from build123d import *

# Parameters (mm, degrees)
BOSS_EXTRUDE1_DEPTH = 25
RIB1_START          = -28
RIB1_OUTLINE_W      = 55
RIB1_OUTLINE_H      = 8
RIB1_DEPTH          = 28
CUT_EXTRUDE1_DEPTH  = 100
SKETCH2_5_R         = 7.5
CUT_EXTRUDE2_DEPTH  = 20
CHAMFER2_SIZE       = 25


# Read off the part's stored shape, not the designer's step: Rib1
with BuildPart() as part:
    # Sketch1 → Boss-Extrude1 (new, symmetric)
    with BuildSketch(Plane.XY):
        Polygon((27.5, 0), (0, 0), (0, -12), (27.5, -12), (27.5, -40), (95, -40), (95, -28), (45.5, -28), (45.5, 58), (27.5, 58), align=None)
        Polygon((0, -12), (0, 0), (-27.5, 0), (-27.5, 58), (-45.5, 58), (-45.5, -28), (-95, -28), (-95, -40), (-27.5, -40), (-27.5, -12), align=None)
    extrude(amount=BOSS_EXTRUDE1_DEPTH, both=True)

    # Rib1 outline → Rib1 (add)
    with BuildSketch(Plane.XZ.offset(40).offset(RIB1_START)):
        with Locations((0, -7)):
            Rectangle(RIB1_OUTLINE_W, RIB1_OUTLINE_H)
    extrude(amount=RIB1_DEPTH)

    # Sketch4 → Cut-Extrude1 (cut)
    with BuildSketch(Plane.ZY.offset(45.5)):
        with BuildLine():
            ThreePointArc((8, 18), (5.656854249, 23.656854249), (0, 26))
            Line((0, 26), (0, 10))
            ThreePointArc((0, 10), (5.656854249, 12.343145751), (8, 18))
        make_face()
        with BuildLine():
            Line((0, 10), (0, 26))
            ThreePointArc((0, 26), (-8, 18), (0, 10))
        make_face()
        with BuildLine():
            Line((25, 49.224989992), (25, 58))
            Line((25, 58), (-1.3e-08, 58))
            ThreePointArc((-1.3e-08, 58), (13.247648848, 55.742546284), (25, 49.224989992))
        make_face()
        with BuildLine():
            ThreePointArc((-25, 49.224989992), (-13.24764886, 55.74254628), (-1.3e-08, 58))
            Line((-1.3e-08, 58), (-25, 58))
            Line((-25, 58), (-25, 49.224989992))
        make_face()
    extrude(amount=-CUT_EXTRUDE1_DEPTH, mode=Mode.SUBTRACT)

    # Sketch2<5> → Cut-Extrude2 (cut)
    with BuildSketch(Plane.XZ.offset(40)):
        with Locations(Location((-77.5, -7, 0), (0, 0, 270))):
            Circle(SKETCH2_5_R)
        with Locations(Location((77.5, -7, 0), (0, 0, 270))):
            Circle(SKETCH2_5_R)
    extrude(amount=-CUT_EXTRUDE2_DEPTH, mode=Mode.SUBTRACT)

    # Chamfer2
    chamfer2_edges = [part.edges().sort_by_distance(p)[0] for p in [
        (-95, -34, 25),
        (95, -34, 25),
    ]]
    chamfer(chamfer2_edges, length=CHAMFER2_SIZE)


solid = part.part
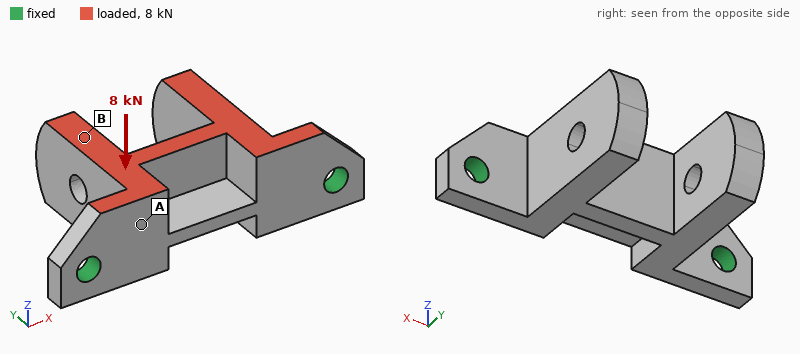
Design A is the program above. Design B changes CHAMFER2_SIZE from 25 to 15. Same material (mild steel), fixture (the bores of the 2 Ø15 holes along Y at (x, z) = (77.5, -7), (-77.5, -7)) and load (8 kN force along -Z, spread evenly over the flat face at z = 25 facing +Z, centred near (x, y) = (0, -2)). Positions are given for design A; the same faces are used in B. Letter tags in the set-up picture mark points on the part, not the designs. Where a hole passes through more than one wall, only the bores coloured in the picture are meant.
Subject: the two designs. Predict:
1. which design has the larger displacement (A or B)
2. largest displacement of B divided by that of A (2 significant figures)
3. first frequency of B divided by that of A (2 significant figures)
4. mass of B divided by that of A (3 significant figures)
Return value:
A
0.92
1.0
1.02
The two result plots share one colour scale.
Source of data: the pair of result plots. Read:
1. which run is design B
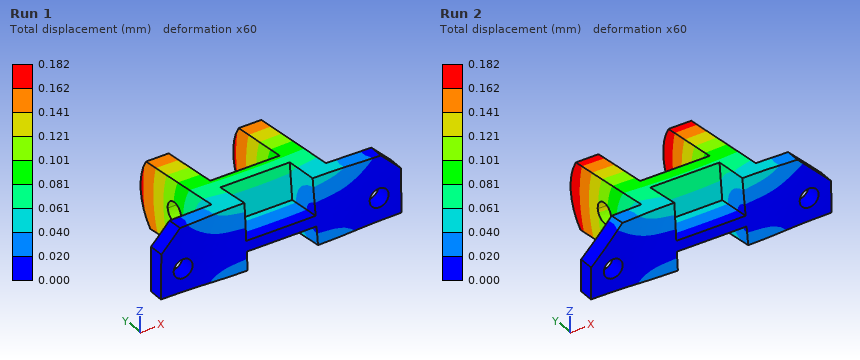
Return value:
Run 1
